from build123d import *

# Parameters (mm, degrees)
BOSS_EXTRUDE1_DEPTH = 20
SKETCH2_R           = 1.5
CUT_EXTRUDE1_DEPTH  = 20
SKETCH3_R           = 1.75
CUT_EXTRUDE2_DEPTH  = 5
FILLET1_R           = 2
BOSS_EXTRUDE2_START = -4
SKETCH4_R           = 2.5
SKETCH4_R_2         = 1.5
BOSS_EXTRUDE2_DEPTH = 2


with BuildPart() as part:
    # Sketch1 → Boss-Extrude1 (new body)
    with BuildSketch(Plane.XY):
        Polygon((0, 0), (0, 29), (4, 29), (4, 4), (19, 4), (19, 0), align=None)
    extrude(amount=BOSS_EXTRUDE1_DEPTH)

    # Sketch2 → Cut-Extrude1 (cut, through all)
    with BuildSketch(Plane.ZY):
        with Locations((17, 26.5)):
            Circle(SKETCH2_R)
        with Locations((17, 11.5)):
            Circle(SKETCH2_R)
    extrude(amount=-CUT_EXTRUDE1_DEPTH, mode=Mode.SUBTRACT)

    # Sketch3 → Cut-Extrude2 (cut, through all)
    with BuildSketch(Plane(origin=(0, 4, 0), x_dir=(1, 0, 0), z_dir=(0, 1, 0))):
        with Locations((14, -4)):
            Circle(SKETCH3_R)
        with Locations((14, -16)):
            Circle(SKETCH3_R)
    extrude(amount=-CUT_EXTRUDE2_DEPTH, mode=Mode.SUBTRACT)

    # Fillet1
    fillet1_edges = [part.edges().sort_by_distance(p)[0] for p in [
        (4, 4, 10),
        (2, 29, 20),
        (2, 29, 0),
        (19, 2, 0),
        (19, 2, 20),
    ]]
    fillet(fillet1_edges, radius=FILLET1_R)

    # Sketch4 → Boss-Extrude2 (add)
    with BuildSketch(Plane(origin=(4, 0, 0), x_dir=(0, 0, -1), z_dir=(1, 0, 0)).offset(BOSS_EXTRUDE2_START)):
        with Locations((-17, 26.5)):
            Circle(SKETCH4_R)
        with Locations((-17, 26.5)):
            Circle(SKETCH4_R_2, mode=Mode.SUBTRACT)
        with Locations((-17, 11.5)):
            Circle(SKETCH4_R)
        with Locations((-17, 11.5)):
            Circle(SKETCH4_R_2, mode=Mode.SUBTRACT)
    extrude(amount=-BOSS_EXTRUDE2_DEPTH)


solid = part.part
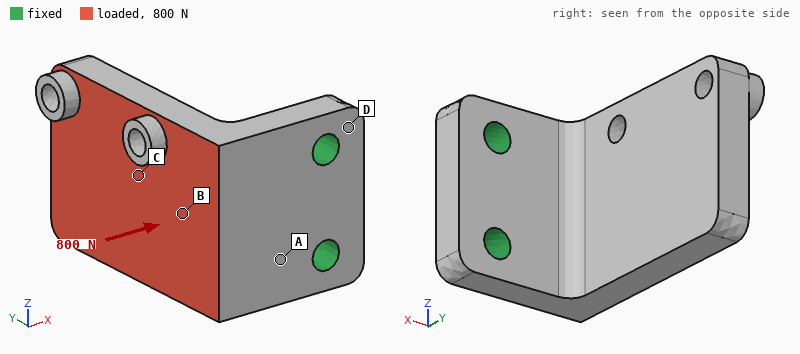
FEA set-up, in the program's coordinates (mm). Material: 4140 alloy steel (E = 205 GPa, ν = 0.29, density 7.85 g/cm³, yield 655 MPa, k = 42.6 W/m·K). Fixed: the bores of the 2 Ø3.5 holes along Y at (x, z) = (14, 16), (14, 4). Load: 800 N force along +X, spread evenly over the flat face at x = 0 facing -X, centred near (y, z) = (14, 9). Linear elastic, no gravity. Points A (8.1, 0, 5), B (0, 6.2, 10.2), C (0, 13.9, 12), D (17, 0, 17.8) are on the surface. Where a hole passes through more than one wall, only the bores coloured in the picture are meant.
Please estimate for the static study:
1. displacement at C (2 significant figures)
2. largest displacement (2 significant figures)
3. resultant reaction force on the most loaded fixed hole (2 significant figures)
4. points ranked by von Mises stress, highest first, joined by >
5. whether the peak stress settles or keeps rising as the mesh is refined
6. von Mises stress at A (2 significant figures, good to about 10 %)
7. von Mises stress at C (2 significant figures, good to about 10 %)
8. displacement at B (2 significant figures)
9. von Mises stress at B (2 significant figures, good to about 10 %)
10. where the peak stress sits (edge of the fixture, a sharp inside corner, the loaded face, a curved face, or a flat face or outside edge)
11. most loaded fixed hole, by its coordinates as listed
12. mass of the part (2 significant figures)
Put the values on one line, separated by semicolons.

0.079 mm; 0.19 mm; 440 N; A > B > C > D; keeps rising; 160 MPa; 55 MPa; 0.043 mm; 120 MPa; edge of the fixture; (14, 4); 27 g
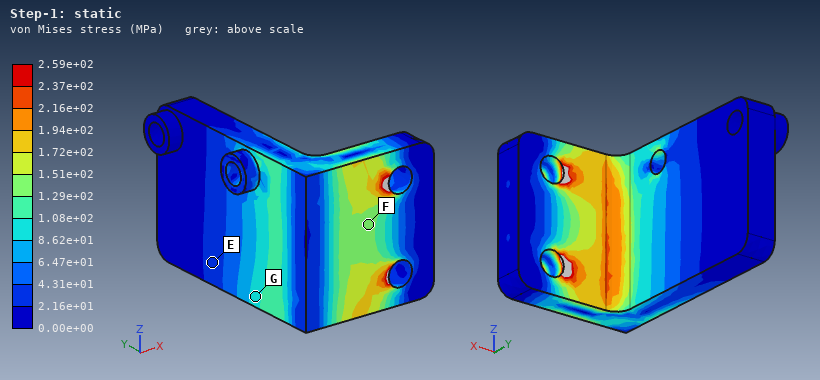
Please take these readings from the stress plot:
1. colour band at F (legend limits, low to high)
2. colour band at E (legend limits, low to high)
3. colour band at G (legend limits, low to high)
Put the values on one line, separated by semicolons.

1.29e+02 to 1.51e+02 MPa; 2.16e+01 to 4.31e+01 MPa; 8.62e+01 to 1.08e+02 MPa
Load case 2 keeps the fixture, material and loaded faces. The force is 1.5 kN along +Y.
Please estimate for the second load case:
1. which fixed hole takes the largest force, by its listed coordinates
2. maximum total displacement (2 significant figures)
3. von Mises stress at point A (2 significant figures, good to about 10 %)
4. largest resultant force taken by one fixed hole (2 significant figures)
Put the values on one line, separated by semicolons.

(14, 4); 0.19 mm; 220 MPa; 800 N
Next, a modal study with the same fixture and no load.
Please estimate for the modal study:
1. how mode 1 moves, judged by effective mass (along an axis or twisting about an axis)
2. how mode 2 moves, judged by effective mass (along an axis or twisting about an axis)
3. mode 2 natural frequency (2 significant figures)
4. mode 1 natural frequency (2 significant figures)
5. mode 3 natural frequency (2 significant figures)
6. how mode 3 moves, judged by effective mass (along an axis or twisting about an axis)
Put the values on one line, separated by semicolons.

along X; along Z; 5500 Hz; 2900 Hz; 11 kHz; along Y
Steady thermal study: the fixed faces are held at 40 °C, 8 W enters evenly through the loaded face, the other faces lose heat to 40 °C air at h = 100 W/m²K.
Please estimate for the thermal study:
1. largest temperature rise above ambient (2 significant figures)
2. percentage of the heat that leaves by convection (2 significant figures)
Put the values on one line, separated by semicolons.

32 K; 38 %
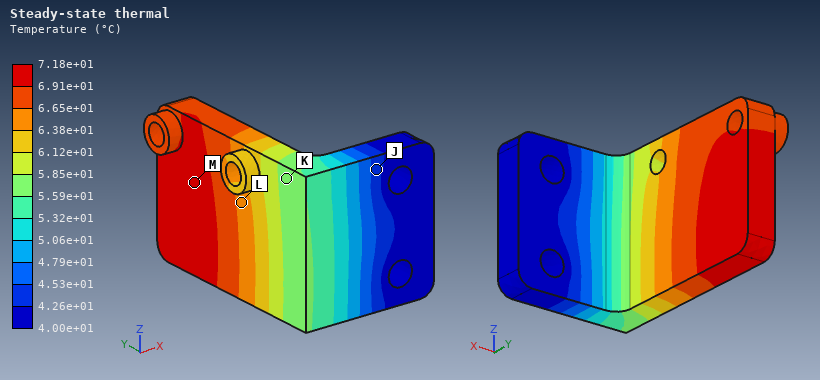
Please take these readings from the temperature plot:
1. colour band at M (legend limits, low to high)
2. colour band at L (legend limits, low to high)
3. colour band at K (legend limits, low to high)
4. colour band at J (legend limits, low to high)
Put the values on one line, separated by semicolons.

6.91e+01 to 7.18e+01 °C; 6.38e+01 to 6.65e+01 °C; 5.59e+01 to 5.85e+01 °C; 4.26e+01 to 4.53e+01 °C
